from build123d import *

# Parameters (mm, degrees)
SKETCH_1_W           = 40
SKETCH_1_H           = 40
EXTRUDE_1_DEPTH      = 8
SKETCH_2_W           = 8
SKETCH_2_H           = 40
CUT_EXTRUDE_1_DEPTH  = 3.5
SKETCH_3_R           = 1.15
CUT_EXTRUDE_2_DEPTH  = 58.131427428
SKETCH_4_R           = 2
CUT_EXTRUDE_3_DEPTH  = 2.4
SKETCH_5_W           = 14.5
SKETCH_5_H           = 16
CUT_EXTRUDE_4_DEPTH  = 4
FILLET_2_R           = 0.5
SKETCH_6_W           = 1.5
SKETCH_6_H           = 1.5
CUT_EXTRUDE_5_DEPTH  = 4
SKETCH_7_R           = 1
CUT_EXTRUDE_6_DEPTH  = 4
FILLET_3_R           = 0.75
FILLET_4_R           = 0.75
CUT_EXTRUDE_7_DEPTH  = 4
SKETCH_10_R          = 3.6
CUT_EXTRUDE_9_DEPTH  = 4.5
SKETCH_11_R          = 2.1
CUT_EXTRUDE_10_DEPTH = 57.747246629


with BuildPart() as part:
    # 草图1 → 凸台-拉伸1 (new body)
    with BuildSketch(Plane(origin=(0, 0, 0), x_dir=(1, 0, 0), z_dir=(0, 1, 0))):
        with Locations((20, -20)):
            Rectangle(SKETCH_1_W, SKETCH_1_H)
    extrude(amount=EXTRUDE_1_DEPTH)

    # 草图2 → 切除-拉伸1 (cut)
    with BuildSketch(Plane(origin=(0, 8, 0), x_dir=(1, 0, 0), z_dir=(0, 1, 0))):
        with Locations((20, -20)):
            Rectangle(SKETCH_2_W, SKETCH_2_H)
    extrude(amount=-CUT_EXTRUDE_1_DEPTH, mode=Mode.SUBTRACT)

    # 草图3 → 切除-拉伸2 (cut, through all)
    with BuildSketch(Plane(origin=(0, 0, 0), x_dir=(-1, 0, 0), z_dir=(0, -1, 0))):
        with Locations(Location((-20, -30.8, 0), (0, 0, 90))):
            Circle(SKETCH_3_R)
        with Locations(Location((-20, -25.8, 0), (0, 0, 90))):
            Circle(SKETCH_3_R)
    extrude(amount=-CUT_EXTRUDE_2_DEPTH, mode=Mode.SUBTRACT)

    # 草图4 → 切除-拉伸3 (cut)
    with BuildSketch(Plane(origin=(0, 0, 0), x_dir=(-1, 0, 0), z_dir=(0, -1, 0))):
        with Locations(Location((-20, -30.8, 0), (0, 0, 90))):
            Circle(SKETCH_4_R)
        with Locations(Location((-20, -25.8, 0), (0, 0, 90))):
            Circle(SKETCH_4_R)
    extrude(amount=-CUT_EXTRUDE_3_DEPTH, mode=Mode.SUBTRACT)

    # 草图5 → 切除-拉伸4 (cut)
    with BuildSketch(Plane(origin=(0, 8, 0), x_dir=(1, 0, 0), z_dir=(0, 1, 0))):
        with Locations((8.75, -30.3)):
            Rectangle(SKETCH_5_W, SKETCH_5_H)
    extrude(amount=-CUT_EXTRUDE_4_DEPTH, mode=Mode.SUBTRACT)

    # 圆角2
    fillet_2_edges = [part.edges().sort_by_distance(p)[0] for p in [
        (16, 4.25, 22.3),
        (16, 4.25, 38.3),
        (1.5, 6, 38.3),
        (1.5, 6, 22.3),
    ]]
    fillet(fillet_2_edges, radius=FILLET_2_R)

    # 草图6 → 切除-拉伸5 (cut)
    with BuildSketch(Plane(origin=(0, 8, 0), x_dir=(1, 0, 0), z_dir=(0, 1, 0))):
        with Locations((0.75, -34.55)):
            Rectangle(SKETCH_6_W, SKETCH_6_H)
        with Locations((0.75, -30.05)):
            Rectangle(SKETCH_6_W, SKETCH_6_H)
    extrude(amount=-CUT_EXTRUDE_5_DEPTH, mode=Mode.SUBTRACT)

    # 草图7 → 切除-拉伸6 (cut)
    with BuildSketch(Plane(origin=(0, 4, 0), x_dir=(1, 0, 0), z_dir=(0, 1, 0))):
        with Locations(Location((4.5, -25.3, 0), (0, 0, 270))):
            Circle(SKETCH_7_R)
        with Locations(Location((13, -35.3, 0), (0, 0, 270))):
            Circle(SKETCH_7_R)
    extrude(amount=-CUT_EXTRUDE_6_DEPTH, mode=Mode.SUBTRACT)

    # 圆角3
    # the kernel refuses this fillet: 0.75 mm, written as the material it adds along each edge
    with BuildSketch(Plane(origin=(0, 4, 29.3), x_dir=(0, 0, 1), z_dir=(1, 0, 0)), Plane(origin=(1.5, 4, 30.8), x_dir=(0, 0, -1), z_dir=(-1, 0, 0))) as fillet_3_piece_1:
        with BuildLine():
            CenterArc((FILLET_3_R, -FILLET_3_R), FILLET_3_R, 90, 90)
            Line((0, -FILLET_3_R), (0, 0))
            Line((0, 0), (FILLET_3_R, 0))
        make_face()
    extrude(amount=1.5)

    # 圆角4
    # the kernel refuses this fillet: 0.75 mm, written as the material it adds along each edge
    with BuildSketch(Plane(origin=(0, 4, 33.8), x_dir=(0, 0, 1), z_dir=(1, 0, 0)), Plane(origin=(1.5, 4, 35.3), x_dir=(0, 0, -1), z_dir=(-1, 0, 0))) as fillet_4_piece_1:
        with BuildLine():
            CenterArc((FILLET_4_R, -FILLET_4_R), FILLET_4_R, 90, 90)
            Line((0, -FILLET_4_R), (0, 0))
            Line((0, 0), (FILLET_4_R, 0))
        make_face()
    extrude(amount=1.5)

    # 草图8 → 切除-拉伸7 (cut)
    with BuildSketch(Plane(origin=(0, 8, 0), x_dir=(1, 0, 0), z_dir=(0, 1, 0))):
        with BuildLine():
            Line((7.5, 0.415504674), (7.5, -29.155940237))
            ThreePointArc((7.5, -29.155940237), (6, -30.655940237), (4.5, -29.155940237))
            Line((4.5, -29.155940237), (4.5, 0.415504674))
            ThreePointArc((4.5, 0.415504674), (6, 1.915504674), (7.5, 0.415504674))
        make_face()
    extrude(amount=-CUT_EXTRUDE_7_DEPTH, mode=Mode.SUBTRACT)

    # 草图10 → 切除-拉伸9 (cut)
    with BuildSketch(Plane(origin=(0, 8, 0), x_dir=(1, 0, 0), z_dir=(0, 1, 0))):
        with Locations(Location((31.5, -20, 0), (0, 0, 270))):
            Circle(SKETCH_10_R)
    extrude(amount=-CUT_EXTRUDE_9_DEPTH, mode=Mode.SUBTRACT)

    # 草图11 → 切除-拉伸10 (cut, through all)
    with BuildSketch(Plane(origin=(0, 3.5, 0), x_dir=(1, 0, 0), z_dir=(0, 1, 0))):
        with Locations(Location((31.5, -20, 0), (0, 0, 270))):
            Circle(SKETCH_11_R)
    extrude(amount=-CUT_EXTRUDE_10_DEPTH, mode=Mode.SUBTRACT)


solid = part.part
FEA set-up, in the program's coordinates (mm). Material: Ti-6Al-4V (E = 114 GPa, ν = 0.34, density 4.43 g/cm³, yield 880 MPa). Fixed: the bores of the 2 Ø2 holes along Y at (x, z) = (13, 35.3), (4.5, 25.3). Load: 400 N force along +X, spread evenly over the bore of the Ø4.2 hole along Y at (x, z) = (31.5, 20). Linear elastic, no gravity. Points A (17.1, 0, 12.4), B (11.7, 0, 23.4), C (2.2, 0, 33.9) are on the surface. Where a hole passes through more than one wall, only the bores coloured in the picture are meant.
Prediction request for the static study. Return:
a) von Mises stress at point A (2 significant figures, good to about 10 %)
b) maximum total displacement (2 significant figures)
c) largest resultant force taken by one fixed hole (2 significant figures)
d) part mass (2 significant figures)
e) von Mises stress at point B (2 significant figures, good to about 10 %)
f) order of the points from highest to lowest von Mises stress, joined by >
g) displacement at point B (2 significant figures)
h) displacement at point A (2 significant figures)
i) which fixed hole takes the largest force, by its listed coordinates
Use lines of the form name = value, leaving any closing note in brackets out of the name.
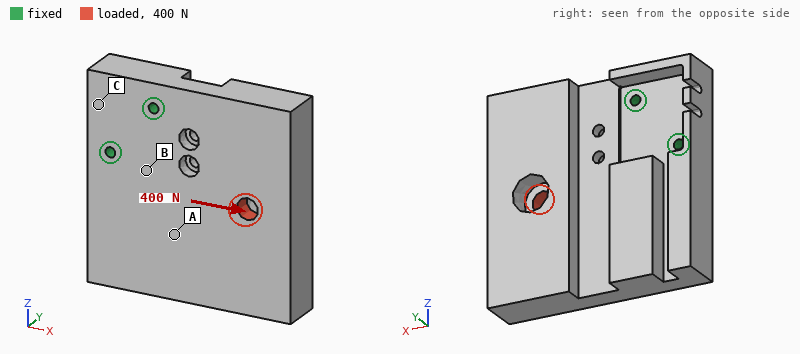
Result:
von Mises stress at point A = 4.1 MPa
maximum total displacement = 6.8 µm
largest resultant force taken by one fixed hole = 460 N
part mass = 45 g
von Mises stress at point B = 11 MPa
order of the points from highest to lowest von Mises stress, joined by > = B > A > C
displacement at point B = 1.1 µm
displacement at point A = 3.2 µm
which fixed hole takes the largest force, by its listed coordinates = (4.5, 25.3)
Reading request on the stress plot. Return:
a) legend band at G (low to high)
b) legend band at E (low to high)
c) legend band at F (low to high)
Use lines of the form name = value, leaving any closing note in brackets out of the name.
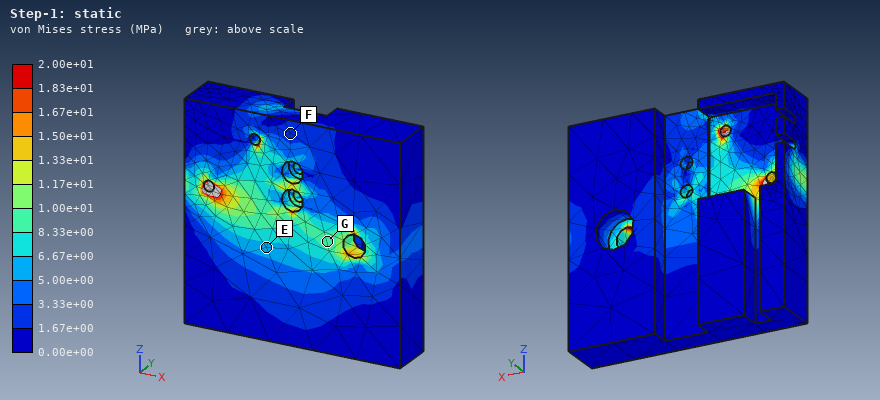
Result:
legend band at G = 8.33e+00 to 1.00e+01 MPa
legend band at E = 5.00e+00 to 6.67e+00 MPa
legend band at F = 1.67e+00 to 3.33e+00 MPa
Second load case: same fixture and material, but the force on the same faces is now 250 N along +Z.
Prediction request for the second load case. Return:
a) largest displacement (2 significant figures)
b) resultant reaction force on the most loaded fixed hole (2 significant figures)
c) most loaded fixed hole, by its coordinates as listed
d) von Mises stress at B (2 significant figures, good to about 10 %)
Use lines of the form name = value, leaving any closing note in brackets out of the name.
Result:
largest displacement = 7.6 µm
resultant reaction force on the most loaded fixed hole = 490 N
most loaded fixed hole, by its coordinates as listed = (13, 35.3)
von Mises stress at B = 7.5 MPa
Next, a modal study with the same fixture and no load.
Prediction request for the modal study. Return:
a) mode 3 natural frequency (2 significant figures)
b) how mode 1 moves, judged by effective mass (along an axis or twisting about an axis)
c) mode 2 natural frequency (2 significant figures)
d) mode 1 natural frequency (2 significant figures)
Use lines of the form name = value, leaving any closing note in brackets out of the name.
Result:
mode 3 natural frequency = 6000 Hz
how mode 1 moves, judged by effective mass = along Y
mode 2 natural frequency = 4500 Hz
mode 1 natural frequency = 1900 Hz
